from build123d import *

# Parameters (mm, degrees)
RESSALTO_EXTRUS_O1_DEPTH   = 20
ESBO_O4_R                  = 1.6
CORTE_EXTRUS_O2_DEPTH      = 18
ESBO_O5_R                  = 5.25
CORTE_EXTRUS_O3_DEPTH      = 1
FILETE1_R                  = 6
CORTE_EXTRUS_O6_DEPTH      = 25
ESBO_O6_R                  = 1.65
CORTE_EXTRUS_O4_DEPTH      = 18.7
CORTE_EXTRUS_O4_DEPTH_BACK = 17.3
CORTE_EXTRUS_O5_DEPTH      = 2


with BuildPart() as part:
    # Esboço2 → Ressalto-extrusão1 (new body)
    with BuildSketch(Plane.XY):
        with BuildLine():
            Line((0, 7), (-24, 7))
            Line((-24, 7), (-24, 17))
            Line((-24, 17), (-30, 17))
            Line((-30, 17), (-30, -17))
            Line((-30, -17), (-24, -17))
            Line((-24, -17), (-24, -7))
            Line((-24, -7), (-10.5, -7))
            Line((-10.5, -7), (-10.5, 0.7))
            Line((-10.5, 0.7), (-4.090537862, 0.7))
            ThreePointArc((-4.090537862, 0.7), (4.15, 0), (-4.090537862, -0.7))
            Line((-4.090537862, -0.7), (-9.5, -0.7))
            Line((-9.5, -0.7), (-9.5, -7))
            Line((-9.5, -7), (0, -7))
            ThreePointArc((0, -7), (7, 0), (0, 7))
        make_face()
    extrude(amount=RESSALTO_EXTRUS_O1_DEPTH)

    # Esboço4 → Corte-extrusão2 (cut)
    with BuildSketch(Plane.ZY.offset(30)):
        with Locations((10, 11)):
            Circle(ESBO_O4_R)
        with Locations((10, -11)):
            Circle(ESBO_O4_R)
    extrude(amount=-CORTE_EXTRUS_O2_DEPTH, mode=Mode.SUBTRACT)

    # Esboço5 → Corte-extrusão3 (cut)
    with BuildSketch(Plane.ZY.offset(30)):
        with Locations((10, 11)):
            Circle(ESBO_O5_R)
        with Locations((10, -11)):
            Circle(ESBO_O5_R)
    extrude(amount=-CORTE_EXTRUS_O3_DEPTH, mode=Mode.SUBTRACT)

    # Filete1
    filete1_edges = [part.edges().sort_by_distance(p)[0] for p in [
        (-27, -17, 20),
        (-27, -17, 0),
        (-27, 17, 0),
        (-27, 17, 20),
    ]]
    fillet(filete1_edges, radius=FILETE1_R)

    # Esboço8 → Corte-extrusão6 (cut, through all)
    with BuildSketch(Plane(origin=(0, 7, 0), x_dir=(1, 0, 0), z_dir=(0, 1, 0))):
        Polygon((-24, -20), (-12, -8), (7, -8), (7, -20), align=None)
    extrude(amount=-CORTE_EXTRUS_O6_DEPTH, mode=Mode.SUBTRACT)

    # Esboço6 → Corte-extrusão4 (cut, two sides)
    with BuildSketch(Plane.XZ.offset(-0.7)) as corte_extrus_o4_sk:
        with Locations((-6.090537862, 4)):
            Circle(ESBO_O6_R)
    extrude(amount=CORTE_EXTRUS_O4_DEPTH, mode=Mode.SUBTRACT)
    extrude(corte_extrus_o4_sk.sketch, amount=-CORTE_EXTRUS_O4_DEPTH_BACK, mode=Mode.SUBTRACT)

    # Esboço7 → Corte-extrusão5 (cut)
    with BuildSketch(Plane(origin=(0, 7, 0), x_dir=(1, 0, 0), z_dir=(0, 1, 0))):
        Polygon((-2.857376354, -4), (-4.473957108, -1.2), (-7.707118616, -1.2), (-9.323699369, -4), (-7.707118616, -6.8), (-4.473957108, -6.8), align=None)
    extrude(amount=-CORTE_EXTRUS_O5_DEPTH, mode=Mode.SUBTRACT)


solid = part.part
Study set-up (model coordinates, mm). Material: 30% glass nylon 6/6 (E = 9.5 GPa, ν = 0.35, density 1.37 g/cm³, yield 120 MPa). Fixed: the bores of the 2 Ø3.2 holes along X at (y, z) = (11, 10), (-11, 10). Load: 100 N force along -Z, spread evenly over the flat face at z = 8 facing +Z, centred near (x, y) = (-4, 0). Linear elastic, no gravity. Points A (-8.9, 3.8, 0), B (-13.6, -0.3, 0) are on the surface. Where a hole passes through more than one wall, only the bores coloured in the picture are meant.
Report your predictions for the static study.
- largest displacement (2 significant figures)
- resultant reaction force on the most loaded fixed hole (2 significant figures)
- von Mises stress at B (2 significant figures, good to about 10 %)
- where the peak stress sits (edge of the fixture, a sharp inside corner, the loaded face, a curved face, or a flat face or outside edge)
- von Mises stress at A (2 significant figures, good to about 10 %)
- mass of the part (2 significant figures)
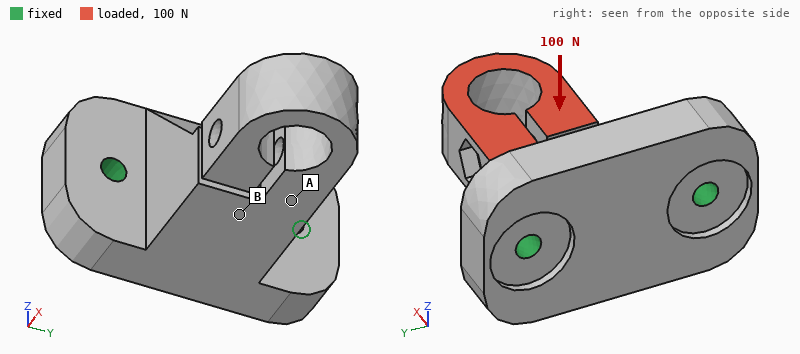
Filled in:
0.62 mm
51 N
5.9 MPa
a curved face
13 MPa
9.9 g
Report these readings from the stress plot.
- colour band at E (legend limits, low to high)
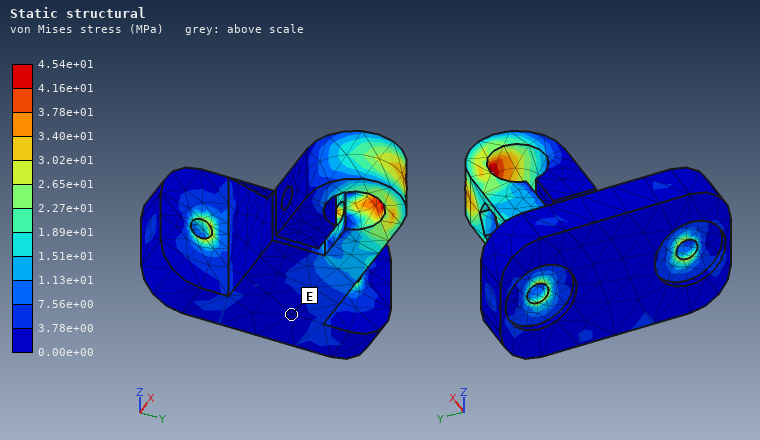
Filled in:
0.00e+00 to 3.78e+00 MPa
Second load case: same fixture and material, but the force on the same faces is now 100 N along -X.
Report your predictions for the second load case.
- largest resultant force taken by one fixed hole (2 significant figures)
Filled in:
52 N
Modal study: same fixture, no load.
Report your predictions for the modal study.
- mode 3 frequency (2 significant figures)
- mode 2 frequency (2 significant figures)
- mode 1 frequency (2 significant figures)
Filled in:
2800 Hz
1800 Hz
1700 Hz
